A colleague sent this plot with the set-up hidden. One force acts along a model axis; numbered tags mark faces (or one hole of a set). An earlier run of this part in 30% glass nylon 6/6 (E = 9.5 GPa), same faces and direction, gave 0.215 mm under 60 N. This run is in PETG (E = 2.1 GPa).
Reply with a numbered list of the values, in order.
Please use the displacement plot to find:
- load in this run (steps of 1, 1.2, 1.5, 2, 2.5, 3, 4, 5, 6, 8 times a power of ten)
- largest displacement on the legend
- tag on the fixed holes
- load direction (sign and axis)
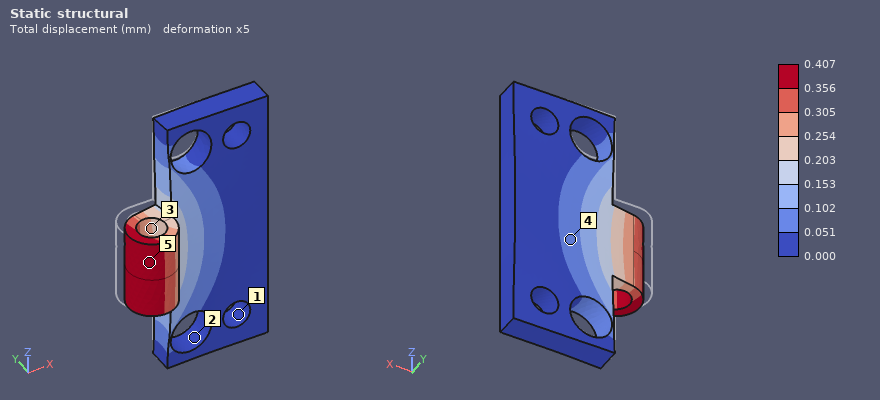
1. 25 N
2. 0.407 mm
3. 1
4. -Y
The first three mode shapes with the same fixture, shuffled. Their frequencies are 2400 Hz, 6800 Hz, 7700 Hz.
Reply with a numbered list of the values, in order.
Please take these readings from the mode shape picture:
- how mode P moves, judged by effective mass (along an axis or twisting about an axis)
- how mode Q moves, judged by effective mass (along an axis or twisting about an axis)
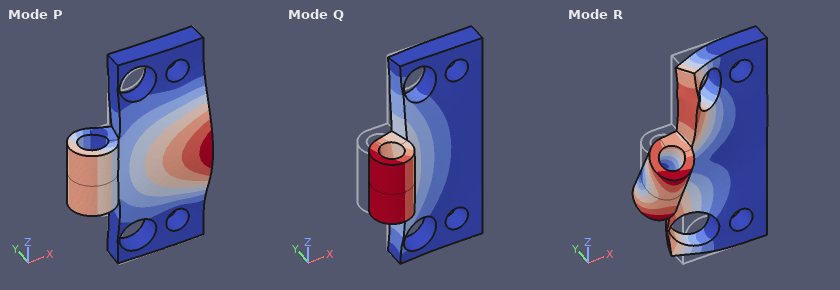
1. along Y
2. along Y
